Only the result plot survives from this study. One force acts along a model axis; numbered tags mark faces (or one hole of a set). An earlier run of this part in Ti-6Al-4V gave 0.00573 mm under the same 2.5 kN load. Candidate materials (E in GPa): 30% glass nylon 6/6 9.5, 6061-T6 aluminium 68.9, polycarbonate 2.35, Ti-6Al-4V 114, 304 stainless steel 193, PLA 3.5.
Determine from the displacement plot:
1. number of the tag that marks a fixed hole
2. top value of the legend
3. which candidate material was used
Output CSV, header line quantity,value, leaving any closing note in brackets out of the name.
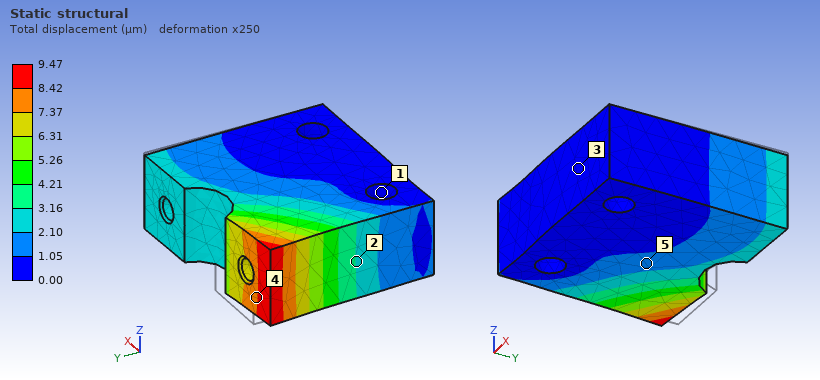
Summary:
quantity,value
number of the tag that marks a fixed hole,1
top value of the legend,9.47 µm
which candidate material was used,6061-T6 aluminium
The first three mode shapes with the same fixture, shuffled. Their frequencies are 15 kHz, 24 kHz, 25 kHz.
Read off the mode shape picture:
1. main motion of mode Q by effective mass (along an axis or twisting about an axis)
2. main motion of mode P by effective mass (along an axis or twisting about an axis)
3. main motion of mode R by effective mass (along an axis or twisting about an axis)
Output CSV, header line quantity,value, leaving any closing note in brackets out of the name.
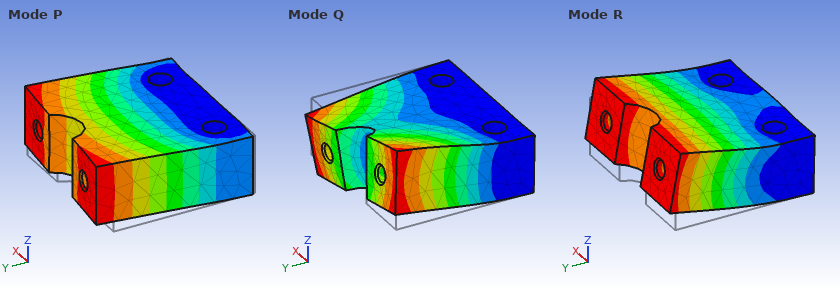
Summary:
quantity,value
main motion of mode Q by effective mass,twisting about Y
main motion of mode P by effective mass,along X
main motion of mode R by effective mass,along Z
